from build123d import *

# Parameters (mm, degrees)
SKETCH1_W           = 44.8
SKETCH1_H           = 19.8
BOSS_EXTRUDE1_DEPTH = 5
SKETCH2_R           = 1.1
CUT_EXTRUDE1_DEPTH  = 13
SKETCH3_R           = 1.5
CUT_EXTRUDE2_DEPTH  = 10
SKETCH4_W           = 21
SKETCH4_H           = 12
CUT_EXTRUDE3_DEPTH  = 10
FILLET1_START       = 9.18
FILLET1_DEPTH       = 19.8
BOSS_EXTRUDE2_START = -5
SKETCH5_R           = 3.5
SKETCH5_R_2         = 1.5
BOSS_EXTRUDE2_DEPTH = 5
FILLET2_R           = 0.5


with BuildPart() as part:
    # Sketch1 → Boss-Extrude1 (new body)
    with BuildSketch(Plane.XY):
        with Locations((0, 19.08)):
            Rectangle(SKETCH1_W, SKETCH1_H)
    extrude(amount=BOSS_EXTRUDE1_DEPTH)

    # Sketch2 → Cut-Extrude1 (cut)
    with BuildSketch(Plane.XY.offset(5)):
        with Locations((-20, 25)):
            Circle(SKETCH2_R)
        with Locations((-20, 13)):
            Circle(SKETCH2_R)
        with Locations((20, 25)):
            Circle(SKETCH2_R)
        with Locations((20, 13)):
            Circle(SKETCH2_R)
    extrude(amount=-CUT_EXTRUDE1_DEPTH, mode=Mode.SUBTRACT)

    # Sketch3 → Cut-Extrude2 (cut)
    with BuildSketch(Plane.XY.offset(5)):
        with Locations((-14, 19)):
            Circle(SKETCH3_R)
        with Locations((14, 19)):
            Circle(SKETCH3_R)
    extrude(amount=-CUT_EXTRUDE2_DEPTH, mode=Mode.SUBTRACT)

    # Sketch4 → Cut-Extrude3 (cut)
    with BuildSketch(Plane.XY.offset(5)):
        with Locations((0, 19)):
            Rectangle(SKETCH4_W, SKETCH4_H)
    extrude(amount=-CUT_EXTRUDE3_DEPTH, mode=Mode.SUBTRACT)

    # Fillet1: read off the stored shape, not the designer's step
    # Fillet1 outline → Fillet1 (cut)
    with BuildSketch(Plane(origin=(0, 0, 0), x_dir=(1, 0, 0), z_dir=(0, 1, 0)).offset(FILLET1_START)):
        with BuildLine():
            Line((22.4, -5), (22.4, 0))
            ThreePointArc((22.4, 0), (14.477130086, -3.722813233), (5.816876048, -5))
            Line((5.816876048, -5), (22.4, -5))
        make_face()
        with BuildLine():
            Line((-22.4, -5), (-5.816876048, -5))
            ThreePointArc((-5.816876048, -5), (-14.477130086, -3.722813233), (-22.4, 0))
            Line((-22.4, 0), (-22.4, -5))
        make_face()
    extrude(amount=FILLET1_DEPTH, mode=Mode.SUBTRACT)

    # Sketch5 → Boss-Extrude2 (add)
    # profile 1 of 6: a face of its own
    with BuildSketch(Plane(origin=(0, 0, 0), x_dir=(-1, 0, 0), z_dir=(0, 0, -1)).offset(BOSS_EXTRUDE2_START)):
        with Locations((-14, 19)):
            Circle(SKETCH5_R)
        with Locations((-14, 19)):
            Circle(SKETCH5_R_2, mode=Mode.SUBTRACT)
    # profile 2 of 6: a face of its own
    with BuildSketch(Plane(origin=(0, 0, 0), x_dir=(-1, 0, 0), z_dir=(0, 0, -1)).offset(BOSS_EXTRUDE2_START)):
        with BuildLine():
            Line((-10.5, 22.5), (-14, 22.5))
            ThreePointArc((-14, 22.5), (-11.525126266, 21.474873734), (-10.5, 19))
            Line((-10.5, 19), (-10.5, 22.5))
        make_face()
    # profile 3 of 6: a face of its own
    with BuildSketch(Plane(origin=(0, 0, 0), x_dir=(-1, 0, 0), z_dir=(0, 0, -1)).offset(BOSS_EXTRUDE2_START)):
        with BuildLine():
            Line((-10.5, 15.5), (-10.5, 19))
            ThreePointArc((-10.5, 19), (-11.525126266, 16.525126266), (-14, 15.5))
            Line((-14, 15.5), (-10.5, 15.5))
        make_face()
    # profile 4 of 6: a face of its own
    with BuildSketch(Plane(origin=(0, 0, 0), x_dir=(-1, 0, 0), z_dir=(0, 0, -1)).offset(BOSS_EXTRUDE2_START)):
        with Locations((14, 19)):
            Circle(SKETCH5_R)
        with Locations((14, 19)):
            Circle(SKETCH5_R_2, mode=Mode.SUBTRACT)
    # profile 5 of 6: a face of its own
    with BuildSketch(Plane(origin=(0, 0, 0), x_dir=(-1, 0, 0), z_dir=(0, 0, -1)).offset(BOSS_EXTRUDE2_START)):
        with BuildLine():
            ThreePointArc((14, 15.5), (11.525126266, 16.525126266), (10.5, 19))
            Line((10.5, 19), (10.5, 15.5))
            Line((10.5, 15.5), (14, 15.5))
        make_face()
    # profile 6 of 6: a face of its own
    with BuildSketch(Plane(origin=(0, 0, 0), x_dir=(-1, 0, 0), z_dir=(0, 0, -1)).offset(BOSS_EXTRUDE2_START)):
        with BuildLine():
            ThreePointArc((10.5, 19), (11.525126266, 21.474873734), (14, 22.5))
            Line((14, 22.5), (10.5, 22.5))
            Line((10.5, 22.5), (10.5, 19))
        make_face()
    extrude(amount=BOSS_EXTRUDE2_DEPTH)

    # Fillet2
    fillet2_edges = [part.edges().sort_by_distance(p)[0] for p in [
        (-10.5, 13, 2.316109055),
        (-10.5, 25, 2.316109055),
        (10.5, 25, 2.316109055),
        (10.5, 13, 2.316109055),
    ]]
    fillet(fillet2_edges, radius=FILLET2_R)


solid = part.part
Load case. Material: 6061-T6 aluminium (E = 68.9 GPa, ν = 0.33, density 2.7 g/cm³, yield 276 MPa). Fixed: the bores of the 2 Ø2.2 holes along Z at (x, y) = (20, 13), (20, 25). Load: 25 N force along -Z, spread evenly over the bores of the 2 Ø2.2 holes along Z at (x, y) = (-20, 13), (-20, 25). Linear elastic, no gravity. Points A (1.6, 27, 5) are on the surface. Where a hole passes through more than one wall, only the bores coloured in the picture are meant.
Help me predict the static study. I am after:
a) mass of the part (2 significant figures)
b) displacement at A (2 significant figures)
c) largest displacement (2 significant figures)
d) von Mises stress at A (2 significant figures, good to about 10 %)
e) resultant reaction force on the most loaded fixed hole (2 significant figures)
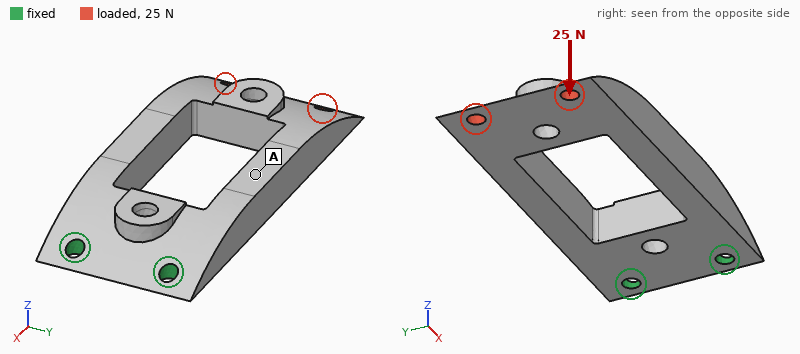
5.8 g
0.080 mm
0.23 mm
16 MPa
13 N
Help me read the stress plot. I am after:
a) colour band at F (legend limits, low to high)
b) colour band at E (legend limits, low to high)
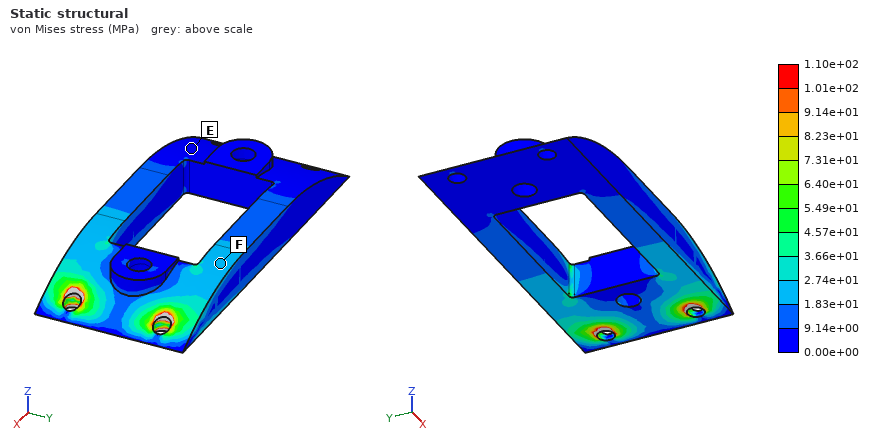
1.83e+01 to 2.74e+01 MPa
0.00e+00 to 9.14e+00 MPa
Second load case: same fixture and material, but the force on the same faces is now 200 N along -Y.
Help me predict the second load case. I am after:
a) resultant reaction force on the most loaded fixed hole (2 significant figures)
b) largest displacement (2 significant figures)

600 N
0.17 mm
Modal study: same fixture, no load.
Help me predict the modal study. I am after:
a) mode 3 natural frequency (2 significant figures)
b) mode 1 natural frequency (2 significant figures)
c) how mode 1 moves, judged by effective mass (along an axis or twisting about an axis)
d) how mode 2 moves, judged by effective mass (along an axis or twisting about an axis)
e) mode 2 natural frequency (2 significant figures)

5500 Hz
1300 Hz
along Z
along Y
3900 Hz
